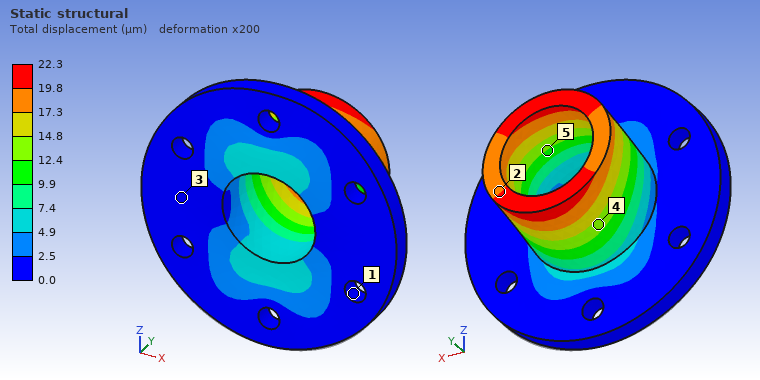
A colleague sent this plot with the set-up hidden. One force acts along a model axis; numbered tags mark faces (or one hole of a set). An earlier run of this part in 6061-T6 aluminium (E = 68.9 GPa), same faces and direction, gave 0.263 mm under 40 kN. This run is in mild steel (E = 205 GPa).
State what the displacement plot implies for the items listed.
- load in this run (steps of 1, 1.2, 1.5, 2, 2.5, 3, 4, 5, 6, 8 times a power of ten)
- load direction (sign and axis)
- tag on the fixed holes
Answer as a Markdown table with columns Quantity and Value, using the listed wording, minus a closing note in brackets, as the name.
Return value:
| Quantity | Value |
|---|---|
| load in this run | 10 kN |
| load direction | +Z |
| tag on the fixed holes | 1 |
